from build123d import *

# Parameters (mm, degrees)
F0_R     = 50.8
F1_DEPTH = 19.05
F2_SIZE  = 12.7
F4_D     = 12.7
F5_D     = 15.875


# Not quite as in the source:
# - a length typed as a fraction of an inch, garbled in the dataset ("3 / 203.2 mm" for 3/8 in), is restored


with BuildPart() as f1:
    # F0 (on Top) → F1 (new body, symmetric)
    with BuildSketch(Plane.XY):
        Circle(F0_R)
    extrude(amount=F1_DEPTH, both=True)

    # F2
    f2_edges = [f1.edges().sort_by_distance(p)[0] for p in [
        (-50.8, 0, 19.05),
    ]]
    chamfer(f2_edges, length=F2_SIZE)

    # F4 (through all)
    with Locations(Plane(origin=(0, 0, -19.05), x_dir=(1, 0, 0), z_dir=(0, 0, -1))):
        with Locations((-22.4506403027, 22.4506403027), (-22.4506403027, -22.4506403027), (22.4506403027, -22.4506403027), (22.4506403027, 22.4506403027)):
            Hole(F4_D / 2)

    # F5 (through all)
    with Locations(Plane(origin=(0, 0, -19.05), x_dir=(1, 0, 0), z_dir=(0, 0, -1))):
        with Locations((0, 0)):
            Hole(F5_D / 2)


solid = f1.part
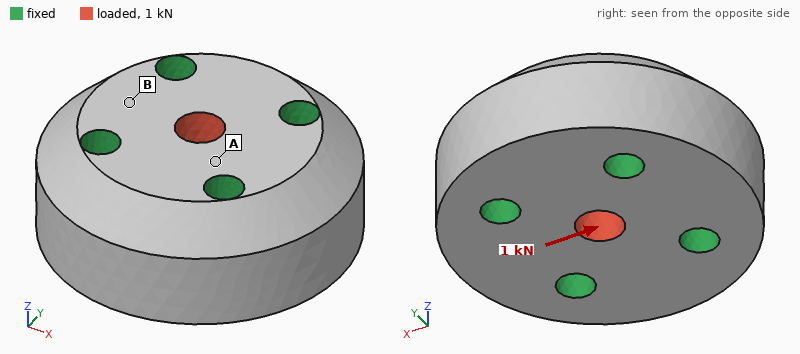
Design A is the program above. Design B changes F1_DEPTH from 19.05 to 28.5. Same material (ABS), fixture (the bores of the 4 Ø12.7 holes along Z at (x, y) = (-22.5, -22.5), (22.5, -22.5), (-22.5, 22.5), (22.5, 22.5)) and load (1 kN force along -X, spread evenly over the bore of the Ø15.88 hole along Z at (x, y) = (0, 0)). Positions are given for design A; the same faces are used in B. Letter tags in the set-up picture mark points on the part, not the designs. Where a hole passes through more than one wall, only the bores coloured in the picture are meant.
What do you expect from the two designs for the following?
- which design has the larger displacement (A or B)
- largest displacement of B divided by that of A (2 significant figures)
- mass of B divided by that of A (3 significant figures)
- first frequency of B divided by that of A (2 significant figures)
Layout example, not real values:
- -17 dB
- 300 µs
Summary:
- A
- 0.68
- 1.54
- 1.1
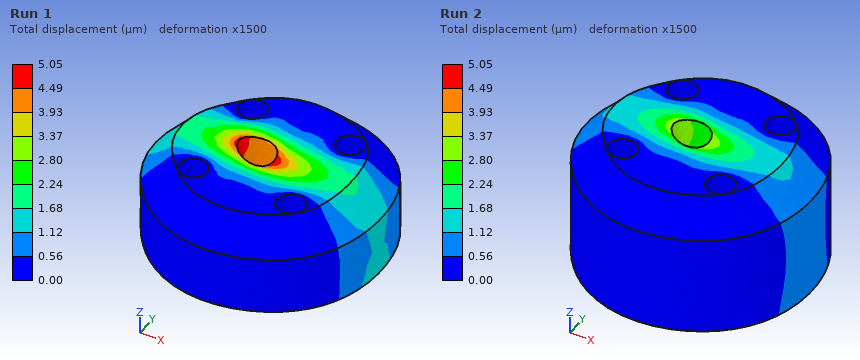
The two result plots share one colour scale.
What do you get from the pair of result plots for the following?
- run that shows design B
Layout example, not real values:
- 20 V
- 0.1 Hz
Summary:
- Run 2
